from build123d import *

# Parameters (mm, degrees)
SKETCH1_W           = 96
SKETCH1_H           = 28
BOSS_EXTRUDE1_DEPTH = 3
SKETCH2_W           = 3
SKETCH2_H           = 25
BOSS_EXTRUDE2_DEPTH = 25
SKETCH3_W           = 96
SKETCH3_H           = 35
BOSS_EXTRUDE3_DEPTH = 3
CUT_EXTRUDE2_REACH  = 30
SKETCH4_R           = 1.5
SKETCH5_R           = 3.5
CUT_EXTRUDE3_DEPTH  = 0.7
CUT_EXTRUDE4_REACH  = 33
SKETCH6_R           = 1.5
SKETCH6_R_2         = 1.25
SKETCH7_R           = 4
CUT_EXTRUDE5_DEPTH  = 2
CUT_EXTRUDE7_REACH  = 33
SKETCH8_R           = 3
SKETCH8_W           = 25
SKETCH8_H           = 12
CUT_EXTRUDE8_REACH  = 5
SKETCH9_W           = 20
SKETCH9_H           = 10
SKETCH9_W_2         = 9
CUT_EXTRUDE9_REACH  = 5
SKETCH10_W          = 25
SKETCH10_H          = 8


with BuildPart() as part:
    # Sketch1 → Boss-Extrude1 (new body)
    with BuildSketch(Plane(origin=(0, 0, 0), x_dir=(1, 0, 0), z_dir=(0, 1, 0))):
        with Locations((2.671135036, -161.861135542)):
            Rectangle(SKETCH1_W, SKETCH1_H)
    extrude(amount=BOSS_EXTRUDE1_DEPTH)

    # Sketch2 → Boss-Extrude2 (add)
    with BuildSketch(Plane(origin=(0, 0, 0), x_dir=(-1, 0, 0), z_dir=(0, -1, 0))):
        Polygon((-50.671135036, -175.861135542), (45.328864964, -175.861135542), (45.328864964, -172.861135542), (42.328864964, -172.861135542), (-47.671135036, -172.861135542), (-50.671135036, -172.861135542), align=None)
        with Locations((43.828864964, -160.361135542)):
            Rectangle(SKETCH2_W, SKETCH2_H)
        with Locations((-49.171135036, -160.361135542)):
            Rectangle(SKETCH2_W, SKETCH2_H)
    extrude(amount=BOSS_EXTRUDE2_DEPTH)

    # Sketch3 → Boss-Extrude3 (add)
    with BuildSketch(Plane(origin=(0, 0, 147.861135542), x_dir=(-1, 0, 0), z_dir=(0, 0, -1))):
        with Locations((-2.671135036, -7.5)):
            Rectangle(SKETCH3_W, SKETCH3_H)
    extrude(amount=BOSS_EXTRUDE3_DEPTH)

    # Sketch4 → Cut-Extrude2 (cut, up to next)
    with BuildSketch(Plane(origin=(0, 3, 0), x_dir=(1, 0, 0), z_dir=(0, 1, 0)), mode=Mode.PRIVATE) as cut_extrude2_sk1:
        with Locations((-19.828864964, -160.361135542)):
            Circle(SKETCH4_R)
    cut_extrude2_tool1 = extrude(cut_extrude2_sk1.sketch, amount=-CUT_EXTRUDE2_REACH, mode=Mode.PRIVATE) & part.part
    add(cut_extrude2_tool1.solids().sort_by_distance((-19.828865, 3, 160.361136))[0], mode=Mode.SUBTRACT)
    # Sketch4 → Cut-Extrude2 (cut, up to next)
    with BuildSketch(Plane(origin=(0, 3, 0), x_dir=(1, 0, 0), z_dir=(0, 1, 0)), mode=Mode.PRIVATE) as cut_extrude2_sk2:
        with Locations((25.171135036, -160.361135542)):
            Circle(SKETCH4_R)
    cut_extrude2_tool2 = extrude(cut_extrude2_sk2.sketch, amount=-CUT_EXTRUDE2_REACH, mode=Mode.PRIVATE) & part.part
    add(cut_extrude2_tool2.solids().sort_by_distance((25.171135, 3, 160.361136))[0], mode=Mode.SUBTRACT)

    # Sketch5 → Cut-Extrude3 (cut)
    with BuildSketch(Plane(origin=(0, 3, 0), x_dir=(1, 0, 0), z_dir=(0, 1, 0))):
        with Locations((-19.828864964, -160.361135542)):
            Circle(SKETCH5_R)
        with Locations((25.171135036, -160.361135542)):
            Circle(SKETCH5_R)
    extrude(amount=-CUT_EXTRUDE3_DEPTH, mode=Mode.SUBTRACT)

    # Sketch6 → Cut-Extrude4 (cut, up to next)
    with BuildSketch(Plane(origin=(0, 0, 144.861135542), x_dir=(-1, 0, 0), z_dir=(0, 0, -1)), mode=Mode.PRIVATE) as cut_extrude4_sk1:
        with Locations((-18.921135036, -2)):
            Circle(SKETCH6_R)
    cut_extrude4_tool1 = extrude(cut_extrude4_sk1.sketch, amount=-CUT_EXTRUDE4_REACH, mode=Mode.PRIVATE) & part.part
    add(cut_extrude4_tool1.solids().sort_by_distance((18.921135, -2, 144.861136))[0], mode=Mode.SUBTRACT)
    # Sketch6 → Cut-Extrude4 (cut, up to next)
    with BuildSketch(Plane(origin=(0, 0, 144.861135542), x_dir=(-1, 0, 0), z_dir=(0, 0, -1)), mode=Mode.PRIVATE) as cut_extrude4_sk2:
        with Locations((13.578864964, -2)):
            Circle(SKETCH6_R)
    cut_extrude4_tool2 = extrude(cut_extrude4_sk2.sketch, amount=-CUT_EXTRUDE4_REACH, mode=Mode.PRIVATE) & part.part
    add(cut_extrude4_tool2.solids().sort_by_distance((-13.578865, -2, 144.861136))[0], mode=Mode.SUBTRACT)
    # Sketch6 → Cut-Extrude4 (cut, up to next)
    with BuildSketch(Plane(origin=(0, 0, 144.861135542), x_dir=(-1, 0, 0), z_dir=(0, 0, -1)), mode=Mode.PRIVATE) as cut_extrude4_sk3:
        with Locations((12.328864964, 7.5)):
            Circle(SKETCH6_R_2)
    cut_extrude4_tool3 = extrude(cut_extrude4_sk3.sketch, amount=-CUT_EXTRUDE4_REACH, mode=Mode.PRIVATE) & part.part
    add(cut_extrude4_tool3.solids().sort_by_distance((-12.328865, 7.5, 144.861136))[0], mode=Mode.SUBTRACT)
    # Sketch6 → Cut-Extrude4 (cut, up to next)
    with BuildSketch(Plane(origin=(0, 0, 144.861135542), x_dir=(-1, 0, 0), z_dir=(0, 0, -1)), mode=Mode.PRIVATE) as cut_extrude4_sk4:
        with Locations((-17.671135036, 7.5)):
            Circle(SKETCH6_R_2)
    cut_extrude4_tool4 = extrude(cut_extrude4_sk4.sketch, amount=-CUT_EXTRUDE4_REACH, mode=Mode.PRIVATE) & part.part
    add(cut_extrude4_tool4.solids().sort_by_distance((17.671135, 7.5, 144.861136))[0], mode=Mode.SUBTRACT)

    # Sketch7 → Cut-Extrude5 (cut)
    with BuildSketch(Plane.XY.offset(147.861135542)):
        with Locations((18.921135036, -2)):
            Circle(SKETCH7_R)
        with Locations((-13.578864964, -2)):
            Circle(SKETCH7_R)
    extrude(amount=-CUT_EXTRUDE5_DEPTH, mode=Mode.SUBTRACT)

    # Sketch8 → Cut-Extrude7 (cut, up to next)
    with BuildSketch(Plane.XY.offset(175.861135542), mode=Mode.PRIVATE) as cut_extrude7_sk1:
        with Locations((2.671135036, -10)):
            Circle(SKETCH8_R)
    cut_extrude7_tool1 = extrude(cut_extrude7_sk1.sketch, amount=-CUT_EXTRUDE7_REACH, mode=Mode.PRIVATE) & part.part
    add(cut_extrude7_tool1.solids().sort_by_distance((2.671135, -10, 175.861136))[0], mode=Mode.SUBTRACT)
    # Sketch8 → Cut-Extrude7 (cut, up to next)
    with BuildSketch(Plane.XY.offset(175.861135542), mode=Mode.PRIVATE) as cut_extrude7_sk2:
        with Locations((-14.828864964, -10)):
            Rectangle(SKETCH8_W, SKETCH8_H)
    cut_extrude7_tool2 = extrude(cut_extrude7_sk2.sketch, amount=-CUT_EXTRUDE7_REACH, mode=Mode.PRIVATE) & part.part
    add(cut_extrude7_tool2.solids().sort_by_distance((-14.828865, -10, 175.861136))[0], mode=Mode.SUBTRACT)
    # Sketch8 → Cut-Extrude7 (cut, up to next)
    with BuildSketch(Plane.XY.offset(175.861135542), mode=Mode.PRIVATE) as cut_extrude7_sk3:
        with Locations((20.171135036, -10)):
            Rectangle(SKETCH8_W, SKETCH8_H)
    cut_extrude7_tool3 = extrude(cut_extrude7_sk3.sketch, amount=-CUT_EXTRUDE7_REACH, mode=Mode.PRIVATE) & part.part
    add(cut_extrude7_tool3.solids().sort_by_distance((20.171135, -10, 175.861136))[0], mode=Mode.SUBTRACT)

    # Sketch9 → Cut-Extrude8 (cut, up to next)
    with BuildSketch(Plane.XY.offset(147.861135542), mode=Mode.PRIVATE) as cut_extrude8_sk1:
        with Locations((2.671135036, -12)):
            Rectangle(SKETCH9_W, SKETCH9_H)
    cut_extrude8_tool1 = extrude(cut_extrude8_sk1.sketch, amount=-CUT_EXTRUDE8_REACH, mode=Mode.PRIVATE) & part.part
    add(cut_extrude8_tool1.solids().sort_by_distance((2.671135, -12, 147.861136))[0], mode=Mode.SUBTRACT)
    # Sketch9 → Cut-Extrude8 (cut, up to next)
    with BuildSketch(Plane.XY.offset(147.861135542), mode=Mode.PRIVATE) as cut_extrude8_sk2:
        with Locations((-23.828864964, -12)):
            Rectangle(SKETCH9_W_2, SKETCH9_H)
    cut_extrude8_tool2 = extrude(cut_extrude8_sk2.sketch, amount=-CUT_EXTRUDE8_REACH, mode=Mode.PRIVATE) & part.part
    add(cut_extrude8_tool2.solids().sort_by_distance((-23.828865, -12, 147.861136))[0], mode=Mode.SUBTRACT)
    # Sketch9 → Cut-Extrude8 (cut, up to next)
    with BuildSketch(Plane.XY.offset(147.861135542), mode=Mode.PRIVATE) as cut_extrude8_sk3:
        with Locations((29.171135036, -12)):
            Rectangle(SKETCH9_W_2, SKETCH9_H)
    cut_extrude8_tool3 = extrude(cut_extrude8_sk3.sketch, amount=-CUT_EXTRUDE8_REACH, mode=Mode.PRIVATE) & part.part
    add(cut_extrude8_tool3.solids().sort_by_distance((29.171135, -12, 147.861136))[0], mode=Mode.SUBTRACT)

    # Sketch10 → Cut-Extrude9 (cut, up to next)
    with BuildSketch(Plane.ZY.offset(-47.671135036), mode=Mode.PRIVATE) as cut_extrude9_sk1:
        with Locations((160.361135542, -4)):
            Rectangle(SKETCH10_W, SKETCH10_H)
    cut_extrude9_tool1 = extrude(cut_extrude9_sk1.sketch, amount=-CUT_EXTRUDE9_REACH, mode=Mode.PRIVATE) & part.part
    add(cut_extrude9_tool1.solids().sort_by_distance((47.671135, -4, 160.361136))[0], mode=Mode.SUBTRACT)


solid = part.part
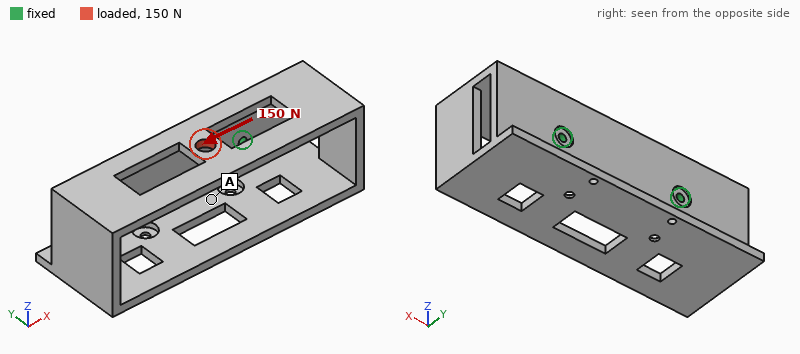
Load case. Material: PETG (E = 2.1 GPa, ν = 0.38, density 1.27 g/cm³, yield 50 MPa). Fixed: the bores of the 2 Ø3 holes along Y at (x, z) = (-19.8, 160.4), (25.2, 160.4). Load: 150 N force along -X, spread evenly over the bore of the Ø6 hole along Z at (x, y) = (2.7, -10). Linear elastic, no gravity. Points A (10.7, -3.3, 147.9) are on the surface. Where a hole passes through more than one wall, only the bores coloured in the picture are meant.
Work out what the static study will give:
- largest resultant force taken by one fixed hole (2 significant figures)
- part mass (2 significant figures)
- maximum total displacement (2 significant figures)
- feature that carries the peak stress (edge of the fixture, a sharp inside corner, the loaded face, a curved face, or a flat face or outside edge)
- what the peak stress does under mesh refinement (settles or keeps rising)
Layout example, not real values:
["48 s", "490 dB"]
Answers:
["95 N", "32 g", "0.49 mm", "edge of the fixture", "keeps rising"]
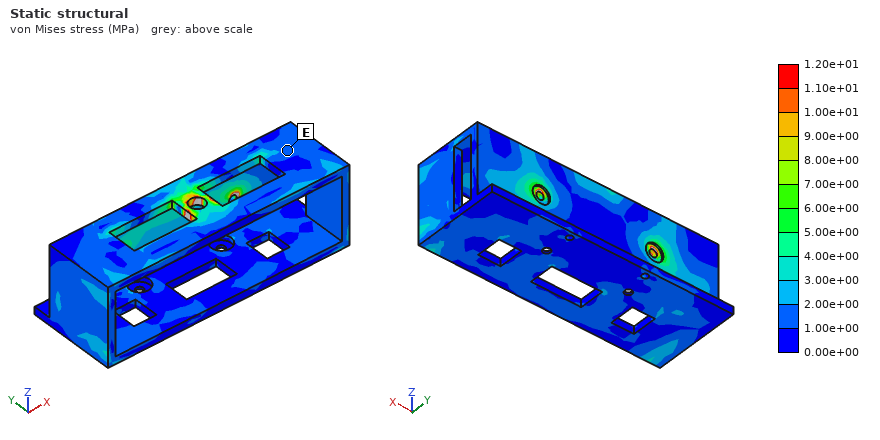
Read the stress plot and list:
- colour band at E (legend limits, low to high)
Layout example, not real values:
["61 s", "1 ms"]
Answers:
["1.00e+00 to 2.00e+00 MPa"]
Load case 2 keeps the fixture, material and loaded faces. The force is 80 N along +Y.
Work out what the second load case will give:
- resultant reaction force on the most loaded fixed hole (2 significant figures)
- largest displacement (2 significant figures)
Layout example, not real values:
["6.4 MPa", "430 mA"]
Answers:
["41 N", "1.1 mm"]
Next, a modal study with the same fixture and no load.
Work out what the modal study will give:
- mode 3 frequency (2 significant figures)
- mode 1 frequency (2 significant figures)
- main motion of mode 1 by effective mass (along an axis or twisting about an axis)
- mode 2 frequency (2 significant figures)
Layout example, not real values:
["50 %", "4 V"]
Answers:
["610 Hz", "310 Hz", "along Z", "470 Hz"]
